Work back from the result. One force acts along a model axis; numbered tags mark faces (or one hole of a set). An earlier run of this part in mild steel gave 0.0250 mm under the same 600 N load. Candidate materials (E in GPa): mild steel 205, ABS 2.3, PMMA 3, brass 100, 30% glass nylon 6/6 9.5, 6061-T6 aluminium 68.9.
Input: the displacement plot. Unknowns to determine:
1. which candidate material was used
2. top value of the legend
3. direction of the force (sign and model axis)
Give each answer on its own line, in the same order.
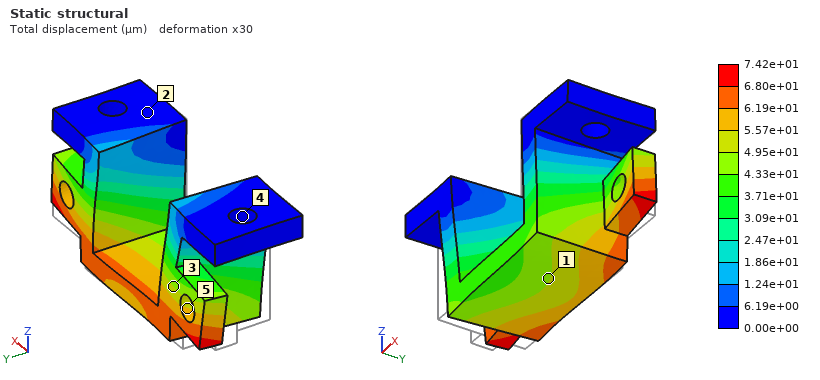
6061-T6 aluminium
7.42e+01 µm
+X
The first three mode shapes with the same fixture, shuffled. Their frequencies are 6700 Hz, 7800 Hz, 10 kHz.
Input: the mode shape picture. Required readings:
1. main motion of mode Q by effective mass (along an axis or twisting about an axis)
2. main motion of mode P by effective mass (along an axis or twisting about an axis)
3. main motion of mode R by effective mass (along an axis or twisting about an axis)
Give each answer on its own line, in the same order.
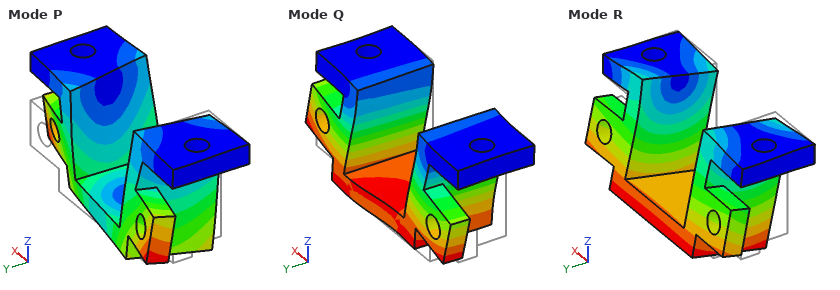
along X
twisting about Z
along Y
